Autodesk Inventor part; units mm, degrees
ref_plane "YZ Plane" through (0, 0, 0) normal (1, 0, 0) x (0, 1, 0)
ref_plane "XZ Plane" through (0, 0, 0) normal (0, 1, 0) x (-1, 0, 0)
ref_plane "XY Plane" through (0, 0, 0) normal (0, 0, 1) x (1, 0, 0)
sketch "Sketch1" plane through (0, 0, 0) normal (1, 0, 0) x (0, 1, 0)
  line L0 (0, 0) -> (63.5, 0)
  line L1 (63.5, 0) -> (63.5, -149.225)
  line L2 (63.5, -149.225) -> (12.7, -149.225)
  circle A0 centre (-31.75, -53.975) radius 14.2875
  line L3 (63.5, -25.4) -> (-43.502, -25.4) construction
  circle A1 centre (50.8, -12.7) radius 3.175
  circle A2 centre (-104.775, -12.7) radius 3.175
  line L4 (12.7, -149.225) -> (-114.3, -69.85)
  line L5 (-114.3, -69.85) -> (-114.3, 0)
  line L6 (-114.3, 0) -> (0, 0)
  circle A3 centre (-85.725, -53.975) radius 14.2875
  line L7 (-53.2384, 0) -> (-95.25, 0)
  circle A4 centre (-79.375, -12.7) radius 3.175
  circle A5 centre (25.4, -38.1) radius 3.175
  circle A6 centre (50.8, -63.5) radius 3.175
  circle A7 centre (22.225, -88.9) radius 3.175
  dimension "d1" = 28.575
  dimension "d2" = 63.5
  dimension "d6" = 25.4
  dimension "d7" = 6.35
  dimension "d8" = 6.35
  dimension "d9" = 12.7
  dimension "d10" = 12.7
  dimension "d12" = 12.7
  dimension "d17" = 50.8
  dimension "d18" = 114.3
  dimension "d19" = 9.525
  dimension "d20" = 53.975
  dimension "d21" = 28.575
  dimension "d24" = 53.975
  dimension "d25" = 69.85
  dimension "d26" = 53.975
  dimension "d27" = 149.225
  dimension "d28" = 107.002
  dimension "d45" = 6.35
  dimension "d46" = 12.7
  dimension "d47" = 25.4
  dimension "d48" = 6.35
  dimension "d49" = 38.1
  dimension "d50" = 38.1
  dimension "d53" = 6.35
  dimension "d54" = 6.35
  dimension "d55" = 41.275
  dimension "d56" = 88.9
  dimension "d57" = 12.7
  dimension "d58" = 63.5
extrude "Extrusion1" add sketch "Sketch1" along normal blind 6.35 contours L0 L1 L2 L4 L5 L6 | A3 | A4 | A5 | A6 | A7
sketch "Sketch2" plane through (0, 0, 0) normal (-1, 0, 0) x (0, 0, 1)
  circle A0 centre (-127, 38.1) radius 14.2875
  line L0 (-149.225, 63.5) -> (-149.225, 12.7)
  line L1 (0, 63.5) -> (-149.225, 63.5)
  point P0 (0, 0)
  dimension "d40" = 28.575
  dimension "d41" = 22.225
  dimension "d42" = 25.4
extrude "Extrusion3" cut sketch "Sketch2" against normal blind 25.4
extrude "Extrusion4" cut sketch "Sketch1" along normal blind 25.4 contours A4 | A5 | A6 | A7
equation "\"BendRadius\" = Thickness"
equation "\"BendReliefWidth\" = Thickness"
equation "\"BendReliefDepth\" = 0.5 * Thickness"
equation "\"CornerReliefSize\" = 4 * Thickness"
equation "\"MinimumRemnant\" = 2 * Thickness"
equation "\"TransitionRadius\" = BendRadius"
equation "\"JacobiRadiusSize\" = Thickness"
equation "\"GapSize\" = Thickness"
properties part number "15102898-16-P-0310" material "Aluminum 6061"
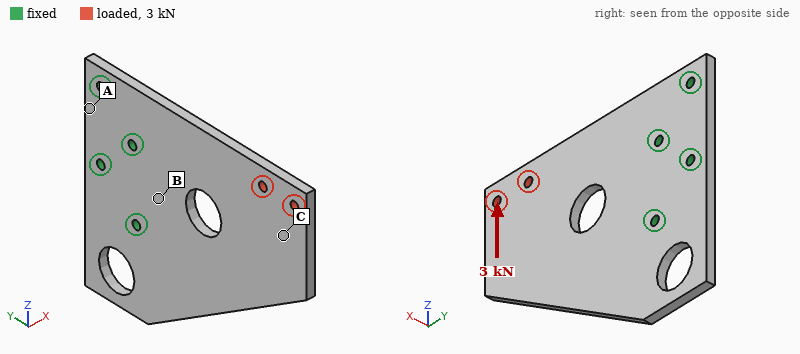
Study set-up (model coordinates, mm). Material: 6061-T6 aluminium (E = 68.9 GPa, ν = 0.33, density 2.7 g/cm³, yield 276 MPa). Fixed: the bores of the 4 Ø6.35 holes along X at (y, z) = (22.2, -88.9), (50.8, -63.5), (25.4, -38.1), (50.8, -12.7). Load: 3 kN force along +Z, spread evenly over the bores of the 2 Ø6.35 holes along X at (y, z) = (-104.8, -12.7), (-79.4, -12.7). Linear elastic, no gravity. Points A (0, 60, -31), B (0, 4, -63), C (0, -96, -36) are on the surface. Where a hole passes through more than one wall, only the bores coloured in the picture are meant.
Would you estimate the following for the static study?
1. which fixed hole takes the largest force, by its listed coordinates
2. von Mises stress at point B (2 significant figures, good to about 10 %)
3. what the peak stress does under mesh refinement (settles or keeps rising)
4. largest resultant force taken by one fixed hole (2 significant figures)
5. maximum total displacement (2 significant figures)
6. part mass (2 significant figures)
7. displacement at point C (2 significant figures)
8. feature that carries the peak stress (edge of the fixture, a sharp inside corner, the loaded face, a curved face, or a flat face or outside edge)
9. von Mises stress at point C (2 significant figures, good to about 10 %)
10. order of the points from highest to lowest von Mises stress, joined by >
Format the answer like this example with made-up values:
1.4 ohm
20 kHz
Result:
(22.2, -88.9)
16 MPa
keeps rising
5.1 kN
95 µm
340 g
76 µm
edge of the fixture
9.7 MPa
B > C > A
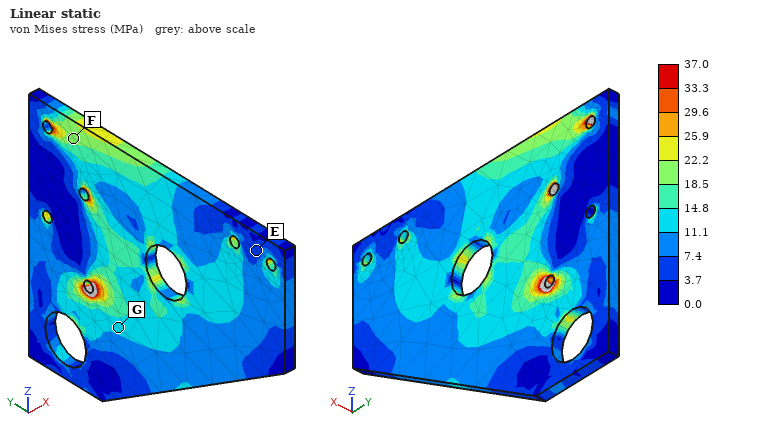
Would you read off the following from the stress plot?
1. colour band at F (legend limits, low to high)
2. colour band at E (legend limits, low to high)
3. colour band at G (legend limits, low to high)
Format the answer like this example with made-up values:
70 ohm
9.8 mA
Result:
18.5 to 22.2 MPa
3.7 to 7.4 MPa
11.1 to 14.8 MPa
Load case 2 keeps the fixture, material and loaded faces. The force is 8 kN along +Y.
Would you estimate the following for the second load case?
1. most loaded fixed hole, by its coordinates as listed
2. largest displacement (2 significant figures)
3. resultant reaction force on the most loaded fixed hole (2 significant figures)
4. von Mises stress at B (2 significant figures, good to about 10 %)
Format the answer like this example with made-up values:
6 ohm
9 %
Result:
(25.4, -38.1)
0.12 mm
4.8 kN
7.5 MPa
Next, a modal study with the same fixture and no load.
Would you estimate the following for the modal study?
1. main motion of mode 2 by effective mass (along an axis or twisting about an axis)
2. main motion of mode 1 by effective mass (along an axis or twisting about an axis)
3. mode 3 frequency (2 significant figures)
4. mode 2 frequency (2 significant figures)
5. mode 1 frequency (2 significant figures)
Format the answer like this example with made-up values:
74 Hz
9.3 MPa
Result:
twisting about Y
along X
1500 Hz
920 Hz
310 Hz
